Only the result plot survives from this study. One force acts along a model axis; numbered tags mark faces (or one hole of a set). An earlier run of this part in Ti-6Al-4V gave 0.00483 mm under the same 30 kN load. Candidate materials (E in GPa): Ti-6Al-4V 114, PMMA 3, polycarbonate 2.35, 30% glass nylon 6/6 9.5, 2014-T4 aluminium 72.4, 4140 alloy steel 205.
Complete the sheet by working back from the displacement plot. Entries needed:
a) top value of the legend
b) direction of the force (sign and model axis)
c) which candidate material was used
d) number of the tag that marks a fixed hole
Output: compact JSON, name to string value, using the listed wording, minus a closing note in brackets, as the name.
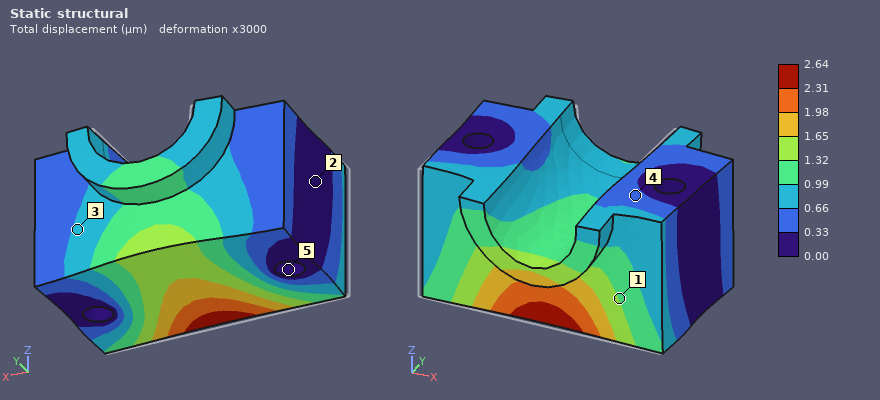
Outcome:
{"top value of the legend": "2.64 µm", "direction of the force": "+Y", "which candidate material was used": "4140 alloy steel", "number of the tag that marks a fixed hole": "5"}
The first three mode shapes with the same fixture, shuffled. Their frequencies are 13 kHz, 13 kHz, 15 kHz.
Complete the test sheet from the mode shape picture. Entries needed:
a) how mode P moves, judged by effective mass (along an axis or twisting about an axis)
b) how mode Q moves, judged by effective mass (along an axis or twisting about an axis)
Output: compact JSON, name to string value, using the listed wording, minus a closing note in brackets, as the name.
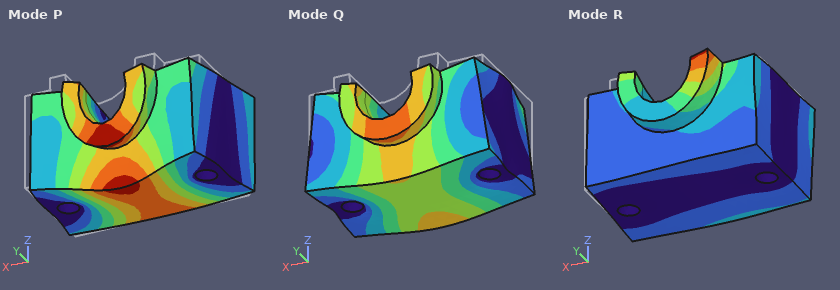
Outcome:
{"how mode P moves, judged by effective mass": "along Y", "how mode Q moves, judged by effective mass": "along Z"}
